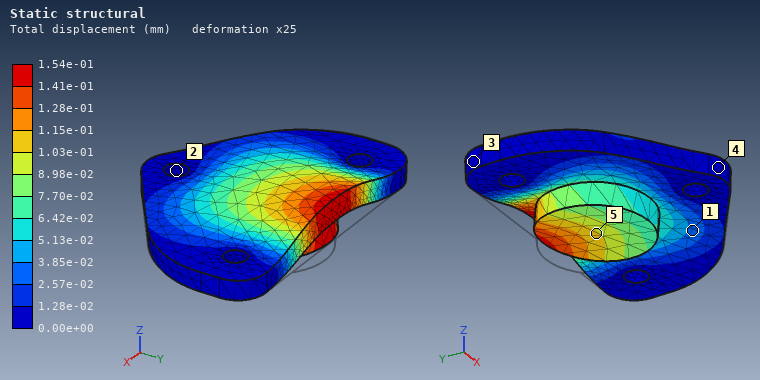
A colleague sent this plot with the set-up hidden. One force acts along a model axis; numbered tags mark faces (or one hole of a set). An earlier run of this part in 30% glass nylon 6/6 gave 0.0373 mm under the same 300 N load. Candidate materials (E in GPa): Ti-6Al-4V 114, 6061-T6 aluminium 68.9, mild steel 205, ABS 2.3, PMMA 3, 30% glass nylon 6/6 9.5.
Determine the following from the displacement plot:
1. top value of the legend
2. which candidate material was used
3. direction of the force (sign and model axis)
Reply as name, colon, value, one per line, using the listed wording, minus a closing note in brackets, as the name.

top value of the legend: 1.54e-01 mm
which candidate material was used: ABS
direction of the force: +Z
